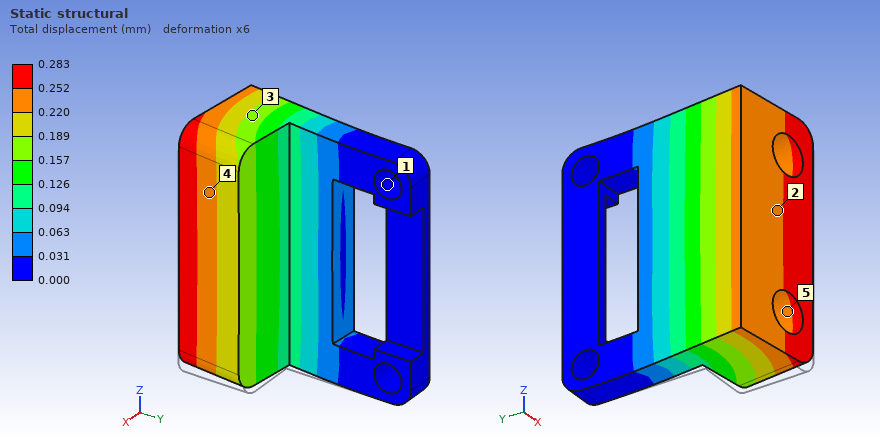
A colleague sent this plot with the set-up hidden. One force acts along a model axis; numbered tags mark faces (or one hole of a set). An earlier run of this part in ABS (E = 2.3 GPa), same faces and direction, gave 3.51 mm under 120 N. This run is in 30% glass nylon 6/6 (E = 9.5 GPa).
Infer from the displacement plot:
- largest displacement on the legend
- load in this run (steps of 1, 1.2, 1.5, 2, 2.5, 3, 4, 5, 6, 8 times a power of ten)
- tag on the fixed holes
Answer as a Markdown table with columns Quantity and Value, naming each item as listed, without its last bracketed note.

| Quantity | Value |
|---|---|
| largest displacement on the legend | 0.283 mm |
| load in this run | 40 N |
| tag on the fixed holes | 1 |
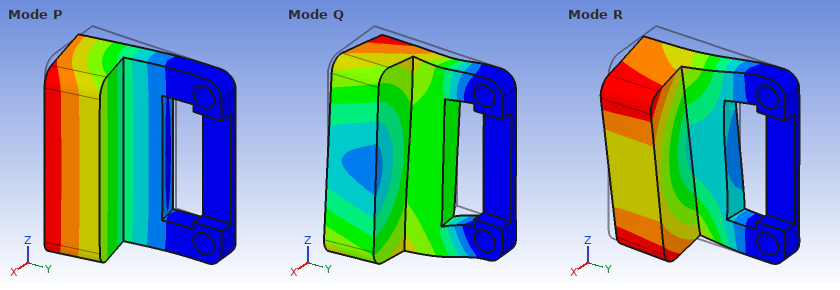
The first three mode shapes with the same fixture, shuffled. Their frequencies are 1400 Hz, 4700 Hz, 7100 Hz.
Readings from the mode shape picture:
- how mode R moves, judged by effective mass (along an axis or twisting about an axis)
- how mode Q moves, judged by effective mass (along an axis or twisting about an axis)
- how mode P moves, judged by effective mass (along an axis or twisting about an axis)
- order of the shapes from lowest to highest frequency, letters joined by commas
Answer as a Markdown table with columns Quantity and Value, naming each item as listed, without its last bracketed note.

| Quantity | Value |
|---|---|
| how mode R moves, judged by effective mass | along Z |
| how mode Q moves, judged by effective mass | along Z |
| how mode P moves, judged by effective mass | along X |
| order of the shapes from lowest to highest frequency, letters joined by commas | P, R, Q |
